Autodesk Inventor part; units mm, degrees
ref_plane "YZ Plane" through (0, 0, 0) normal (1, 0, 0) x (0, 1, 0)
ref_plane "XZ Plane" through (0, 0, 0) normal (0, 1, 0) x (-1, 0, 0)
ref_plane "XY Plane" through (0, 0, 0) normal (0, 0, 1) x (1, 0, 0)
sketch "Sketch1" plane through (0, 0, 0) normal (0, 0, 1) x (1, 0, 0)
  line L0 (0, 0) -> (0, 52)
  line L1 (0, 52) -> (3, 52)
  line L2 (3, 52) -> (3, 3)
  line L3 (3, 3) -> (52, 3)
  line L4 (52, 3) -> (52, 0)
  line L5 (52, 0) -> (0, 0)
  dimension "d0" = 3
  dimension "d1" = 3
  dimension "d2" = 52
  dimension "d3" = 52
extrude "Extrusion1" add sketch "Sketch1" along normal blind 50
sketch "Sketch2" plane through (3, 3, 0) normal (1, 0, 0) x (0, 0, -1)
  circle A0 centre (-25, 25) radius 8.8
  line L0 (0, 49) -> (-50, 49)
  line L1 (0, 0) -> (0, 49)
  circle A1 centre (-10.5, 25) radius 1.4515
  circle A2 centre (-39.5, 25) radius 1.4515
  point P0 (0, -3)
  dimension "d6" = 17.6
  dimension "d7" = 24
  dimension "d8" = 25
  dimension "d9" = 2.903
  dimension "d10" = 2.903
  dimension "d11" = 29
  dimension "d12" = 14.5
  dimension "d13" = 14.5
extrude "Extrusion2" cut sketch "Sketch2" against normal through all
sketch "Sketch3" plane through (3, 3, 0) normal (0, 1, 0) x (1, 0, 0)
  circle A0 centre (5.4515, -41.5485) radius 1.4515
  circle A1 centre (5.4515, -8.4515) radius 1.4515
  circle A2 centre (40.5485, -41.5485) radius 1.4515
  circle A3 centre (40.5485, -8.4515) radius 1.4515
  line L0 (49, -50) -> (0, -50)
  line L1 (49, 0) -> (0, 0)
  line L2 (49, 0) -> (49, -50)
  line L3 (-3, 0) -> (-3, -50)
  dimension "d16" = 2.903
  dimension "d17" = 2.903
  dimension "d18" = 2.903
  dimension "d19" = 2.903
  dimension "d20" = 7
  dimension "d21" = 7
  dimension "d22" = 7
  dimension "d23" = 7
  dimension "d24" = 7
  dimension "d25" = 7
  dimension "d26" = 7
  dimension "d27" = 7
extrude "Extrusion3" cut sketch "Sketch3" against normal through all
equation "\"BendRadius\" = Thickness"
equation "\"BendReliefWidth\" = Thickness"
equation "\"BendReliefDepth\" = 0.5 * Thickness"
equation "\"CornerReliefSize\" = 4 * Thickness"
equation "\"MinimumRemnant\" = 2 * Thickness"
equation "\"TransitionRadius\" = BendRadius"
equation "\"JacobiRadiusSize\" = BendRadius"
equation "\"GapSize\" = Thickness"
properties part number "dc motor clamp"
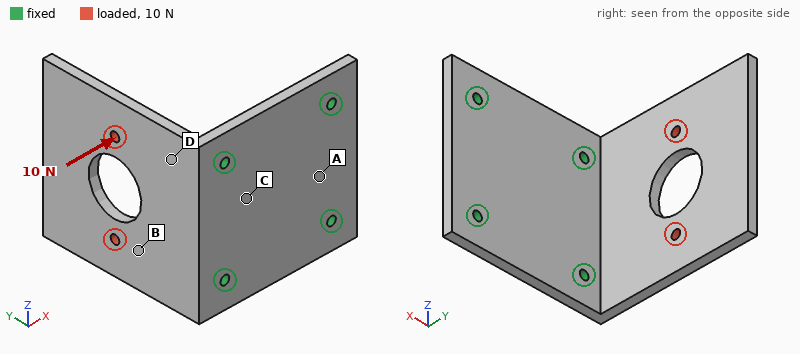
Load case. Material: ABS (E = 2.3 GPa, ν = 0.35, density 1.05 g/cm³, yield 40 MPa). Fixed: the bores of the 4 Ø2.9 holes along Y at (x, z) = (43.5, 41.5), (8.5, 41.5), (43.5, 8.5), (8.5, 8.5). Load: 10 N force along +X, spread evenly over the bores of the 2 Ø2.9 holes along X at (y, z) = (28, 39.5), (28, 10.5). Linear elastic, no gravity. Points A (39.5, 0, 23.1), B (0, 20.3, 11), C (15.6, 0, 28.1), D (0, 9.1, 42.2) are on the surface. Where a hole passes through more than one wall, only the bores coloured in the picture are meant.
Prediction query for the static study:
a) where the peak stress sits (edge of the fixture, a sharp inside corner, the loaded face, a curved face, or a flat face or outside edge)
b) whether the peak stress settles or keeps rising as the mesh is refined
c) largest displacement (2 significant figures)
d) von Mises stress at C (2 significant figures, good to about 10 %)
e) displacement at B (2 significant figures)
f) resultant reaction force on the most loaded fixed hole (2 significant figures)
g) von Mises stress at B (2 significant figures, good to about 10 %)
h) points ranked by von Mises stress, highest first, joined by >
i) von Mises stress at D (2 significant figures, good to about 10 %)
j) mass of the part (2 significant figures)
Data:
edge of the fixture
keeps rising
0.91 mm
0.77 MPa
0.27 mm
4.1 N
1.3 MPa
D > B > C > A
2.4 MPa
15 g
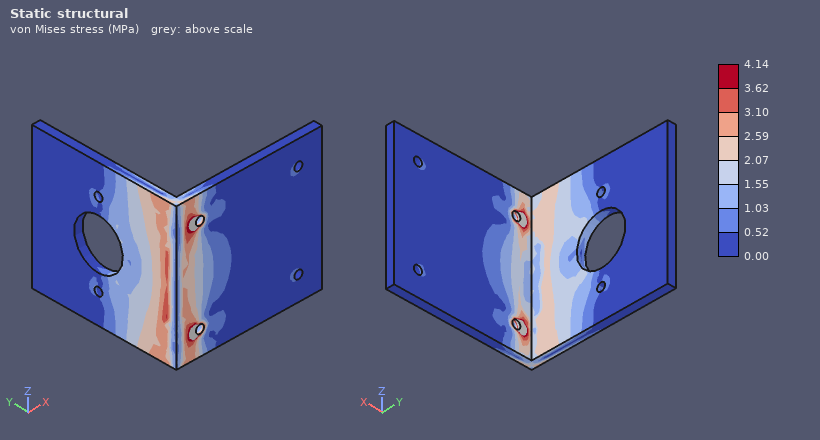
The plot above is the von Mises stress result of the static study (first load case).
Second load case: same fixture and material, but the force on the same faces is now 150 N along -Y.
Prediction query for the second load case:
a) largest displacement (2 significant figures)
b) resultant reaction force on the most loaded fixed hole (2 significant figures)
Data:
0.90 mm
79 N
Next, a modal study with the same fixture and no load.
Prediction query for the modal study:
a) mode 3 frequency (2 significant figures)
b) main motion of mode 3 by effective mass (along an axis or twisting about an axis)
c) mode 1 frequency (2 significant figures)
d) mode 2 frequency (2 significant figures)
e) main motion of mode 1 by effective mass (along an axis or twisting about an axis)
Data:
1200 Hz
along Z
230 Hz
580 Hz
along X
